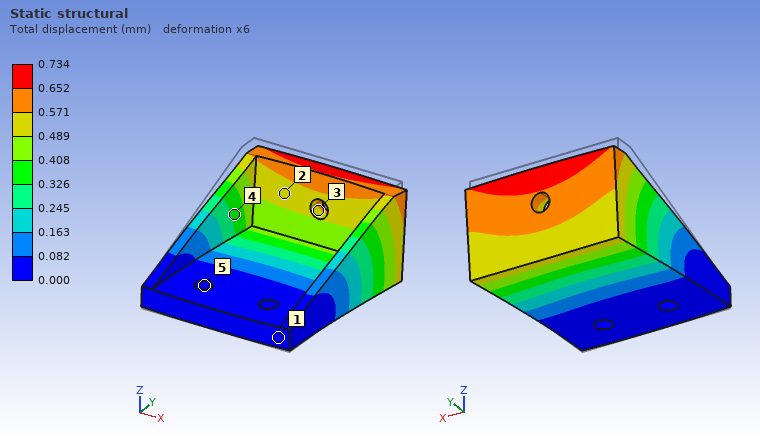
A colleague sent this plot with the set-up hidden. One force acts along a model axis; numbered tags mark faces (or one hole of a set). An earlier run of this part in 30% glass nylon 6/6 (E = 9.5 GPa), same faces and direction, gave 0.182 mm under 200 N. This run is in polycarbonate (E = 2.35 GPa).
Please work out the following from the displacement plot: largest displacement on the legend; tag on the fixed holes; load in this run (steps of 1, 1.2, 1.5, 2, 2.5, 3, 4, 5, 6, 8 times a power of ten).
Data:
0.734 mm
5
200 N
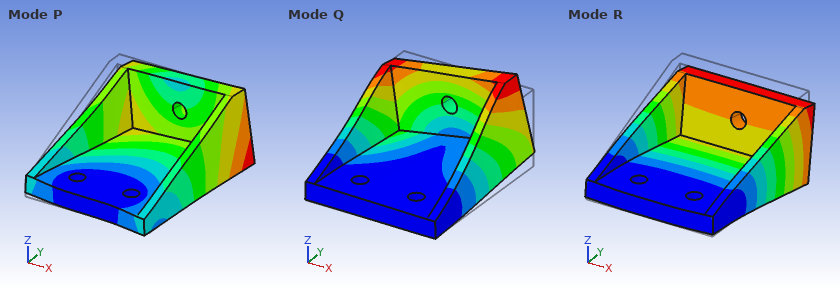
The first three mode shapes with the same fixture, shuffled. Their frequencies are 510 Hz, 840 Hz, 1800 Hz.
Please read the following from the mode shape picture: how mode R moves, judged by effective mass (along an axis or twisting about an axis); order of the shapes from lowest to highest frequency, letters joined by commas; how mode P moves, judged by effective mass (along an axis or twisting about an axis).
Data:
along Z
R, Q, P
along X
